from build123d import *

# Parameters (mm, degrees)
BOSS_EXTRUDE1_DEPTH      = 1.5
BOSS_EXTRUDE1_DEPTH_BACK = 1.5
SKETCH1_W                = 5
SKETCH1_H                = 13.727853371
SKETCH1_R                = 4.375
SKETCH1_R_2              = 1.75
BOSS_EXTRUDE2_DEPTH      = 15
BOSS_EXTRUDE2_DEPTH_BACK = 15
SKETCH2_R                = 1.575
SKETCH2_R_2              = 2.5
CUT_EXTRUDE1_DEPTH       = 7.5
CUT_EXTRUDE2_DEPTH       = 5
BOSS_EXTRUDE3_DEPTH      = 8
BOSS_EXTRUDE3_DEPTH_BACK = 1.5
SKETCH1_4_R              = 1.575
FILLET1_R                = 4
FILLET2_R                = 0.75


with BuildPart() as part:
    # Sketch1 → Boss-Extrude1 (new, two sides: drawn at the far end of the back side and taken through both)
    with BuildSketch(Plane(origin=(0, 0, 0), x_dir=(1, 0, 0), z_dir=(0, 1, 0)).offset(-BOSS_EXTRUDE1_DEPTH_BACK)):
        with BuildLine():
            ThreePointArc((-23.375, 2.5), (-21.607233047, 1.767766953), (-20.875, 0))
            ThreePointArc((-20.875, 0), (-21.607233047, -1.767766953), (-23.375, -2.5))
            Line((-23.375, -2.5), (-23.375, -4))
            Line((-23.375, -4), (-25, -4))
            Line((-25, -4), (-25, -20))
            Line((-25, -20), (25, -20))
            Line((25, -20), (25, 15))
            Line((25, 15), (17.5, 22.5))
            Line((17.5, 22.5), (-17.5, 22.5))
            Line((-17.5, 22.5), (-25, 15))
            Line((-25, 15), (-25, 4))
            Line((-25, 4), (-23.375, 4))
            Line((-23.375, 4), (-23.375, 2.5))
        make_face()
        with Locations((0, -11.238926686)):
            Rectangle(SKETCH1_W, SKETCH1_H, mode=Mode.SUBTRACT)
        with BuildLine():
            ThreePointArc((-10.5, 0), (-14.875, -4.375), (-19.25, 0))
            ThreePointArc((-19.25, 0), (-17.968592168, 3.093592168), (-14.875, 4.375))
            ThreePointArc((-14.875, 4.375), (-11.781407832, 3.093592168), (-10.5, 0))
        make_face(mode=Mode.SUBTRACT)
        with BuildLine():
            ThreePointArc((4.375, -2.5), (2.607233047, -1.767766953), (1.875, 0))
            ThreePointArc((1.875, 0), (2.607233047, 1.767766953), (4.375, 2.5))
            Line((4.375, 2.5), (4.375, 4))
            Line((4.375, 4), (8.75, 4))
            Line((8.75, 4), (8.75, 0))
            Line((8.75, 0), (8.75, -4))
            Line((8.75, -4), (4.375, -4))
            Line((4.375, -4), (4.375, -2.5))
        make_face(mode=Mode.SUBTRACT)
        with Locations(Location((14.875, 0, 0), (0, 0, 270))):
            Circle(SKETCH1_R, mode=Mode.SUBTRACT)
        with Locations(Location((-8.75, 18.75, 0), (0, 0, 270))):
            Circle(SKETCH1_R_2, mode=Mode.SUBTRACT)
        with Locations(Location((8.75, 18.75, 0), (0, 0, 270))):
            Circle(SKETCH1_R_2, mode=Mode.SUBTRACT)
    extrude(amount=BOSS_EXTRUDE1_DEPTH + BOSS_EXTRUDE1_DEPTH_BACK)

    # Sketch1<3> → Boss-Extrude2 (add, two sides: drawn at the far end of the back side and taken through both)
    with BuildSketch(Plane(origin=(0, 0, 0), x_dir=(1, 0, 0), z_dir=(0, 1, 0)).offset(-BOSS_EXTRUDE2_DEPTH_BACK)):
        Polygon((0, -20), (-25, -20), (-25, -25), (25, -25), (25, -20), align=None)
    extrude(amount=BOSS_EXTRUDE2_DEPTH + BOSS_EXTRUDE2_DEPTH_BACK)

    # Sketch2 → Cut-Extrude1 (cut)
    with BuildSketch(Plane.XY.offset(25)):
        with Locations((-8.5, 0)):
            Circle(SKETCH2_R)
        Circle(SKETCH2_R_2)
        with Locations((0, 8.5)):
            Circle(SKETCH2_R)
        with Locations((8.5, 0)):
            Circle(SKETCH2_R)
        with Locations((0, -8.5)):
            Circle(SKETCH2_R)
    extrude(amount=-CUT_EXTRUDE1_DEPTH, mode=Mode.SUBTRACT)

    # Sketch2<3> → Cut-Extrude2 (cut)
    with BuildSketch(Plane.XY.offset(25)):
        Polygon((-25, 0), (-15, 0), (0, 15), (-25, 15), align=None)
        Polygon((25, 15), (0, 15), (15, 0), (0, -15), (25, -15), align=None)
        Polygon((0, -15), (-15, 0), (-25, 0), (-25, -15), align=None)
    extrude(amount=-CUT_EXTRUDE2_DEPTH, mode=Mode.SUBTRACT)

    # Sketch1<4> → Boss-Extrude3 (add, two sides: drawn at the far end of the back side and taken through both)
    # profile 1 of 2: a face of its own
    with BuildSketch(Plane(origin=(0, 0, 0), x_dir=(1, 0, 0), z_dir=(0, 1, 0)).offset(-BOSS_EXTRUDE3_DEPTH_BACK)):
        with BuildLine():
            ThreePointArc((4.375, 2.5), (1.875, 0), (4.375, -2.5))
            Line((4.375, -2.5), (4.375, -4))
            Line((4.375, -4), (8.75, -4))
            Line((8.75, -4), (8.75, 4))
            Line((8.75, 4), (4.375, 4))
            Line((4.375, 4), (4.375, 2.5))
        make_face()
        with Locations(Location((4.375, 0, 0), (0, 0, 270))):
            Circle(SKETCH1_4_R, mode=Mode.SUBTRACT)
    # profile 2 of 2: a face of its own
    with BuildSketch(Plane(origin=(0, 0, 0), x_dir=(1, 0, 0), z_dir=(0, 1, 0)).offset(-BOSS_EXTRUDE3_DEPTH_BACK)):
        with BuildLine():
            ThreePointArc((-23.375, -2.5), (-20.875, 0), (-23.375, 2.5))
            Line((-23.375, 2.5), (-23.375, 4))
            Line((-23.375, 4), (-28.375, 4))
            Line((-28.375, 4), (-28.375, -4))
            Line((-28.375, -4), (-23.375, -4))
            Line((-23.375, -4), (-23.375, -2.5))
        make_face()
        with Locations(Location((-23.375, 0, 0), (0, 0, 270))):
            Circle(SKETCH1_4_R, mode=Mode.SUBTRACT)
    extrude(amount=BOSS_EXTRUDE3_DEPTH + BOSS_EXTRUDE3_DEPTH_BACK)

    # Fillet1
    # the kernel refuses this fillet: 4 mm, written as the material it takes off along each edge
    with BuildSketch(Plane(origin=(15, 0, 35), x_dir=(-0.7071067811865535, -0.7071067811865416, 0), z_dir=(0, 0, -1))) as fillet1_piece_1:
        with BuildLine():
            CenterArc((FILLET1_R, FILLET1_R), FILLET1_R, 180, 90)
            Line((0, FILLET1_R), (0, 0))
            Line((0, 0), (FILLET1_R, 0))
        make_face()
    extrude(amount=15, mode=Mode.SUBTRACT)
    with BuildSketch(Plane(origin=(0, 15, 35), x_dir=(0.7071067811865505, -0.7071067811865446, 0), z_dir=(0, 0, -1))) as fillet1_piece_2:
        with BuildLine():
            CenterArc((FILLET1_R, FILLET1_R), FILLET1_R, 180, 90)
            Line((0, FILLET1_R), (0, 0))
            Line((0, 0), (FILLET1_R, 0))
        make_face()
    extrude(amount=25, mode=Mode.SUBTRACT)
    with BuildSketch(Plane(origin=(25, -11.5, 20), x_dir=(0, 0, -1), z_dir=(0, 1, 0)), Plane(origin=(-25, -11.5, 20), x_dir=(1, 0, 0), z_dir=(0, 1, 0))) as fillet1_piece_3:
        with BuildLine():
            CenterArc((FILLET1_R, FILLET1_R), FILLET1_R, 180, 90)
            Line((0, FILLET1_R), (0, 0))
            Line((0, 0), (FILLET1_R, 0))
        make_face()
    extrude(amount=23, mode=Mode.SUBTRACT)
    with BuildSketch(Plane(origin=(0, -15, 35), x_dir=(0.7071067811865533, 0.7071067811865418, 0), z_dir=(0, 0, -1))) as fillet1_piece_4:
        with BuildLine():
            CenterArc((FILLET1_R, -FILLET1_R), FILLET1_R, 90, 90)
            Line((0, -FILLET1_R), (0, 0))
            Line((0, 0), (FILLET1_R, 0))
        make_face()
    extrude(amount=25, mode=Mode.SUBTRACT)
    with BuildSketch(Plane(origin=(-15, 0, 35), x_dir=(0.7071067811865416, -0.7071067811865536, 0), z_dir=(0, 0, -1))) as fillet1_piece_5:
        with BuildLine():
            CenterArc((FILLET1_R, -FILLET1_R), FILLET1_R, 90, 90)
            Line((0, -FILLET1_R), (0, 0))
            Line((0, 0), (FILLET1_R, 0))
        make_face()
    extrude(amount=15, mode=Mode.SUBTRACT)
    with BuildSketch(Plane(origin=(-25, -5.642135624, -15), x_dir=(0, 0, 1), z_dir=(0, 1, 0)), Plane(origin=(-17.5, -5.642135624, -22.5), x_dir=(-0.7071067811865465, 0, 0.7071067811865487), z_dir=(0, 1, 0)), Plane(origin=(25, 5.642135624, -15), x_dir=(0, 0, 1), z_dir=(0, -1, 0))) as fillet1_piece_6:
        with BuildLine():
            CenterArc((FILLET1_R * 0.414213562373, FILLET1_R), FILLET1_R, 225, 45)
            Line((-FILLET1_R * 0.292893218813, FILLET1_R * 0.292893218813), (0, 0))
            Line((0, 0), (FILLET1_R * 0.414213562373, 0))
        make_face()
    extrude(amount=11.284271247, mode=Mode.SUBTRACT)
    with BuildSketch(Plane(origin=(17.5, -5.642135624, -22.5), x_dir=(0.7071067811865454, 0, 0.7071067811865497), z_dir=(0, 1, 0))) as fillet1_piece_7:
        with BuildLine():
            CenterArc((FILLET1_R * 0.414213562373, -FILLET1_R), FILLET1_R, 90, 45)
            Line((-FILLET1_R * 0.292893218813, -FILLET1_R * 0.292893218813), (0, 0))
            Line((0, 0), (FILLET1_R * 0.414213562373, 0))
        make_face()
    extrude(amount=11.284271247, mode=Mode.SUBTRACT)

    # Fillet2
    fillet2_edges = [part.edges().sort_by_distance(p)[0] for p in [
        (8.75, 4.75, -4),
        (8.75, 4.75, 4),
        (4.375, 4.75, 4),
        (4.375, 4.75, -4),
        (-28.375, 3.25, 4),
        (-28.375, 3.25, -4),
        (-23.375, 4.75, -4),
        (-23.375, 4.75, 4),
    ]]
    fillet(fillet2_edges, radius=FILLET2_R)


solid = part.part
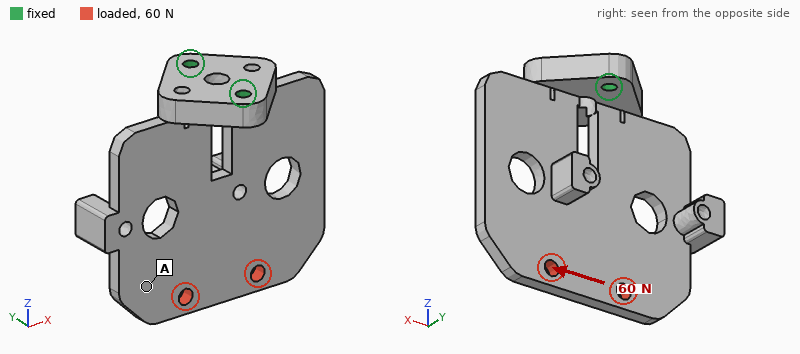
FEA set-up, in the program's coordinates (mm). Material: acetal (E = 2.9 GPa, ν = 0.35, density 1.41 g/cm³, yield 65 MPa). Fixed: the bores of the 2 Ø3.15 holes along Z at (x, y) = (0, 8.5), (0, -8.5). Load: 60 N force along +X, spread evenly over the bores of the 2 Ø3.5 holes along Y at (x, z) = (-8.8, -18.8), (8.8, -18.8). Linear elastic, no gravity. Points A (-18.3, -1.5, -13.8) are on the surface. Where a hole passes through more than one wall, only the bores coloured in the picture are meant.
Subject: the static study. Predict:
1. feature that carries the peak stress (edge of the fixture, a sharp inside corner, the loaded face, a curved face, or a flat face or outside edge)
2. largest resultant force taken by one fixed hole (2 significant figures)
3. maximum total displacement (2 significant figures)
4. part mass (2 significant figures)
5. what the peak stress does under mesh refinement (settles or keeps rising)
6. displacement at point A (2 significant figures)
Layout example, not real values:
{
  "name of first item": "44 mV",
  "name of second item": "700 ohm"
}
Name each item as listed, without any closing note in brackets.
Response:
{
  "feature that carries the peak stress": "edge of the fixture",
  "largest resultant force taken by one fixed hole": "30 N",
  "maximum total displacement": "0.90 mm",
  "part mass": "11 g",
  "what the peak stress does under mesh refinement": "keeps rising",
  "displacement at point A": "0.77 mm"
}
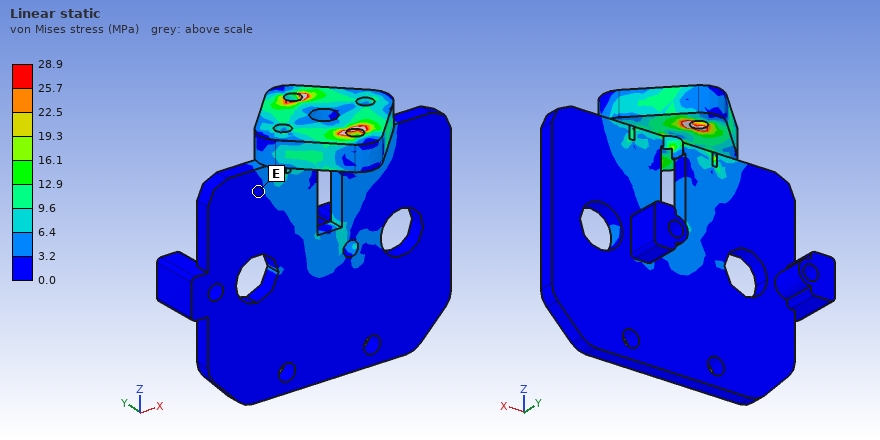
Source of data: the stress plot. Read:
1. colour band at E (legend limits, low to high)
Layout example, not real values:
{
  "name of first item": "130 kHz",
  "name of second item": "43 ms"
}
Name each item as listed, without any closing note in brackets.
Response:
{
  "colour band at E": "0.0 to 3.2 MPa"
}
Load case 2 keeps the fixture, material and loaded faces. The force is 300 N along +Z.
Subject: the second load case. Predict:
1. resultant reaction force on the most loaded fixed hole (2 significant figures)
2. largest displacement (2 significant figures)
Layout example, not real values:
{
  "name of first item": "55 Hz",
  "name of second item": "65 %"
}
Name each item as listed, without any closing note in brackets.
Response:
{
  "resultant reaction force on the most loaded fixed hole": "150 N",
  "largest displacement": "0.12 mm"
}
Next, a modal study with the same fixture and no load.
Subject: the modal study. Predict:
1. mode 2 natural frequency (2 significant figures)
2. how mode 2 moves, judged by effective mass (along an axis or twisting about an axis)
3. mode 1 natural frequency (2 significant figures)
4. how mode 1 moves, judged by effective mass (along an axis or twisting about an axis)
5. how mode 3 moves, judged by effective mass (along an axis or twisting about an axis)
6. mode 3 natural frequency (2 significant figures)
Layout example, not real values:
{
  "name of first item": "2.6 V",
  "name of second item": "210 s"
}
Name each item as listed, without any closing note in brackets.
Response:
{
  "mode 2 natural frequency": "580 Hz",
  "how mode 2 moves, judged by effective mass": "twisting about Z",
  "mode 1 natural frequency": "280 Hz",
  "how mode 1 moves, judged by effective mass": "along Y",
  "how mode 3 moves, judged by effective mass": "along X",
  "mode 3 natural frequency": "650 Hz"
}
